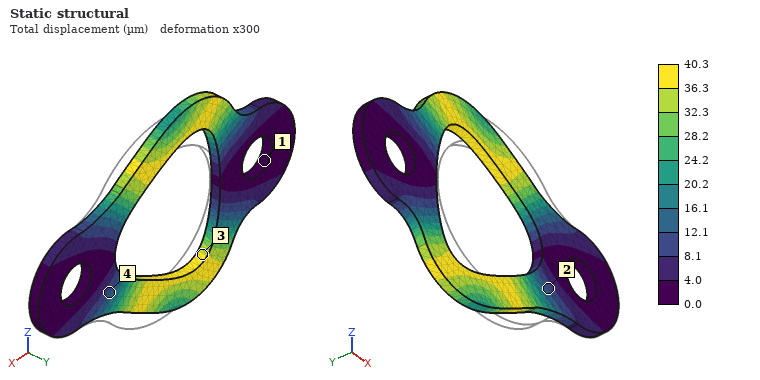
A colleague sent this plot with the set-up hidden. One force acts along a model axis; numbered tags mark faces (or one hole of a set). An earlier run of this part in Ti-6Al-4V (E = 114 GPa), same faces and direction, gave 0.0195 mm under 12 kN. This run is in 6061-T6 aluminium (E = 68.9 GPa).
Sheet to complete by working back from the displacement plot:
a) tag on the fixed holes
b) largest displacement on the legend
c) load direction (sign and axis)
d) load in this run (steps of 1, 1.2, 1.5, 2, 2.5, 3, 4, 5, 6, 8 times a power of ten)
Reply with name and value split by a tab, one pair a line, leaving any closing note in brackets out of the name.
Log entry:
tag on the fixed holes	1
largest displacement on the legend	40.3 µm
load direction	-X
load in this run	15 kN
